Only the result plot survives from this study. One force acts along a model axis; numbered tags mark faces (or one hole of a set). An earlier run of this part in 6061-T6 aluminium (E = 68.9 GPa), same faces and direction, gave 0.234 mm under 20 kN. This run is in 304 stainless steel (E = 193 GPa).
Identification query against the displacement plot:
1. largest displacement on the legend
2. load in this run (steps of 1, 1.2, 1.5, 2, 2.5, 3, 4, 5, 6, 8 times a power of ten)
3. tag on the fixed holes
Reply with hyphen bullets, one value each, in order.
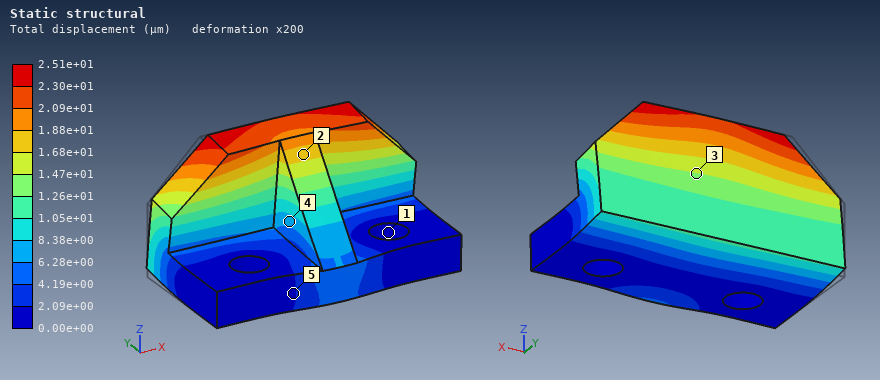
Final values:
- 2.51e+01 µm
- 6 kN
- 1
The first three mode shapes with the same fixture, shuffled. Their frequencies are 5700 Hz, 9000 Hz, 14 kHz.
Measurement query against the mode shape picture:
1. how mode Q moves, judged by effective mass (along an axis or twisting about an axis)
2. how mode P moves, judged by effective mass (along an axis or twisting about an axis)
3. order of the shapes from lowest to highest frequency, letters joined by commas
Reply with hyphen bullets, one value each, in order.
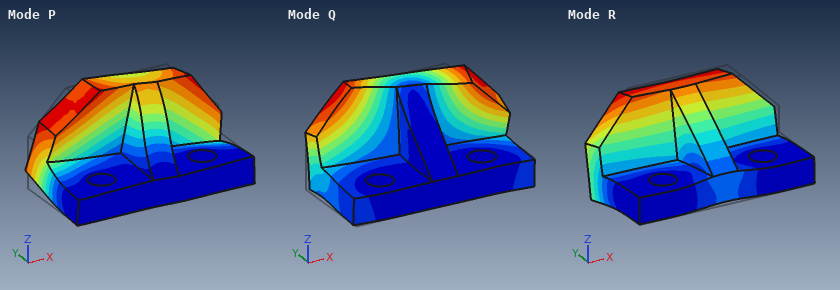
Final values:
- along X
- along X
- R, P, Q
